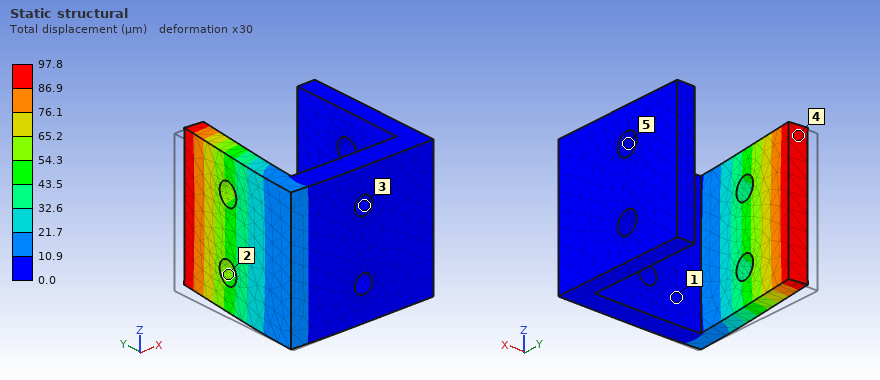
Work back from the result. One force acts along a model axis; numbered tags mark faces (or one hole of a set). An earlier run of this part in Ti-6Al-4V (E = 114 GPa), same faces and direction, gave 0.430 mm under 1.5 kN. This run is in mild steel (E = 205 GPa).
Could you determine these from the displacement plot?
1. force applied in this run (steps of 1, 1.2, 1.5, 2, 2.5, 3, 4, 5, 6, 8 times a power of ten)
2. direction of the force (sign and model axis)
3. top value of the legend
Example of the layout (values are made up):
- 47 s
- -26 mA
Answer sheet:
- 600 N
- +X
- 97.8 µm
